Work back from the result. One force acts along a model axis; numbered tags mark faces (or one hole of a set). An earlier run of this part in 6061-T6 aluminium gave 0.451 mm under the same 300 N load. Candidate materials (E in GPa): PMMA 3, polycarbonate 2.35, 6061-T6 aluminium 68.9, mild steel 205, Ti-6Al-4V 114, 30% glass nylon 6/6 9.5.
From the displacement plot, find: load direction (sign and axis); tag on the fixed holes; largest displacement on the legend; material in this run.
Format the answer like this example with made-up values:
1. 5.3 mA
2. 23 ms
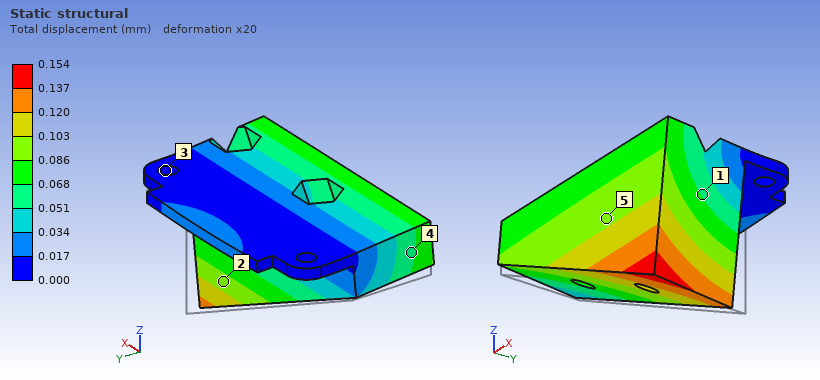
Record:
1. -Y
2. 3
3. 0.154 mm
4. mild steel
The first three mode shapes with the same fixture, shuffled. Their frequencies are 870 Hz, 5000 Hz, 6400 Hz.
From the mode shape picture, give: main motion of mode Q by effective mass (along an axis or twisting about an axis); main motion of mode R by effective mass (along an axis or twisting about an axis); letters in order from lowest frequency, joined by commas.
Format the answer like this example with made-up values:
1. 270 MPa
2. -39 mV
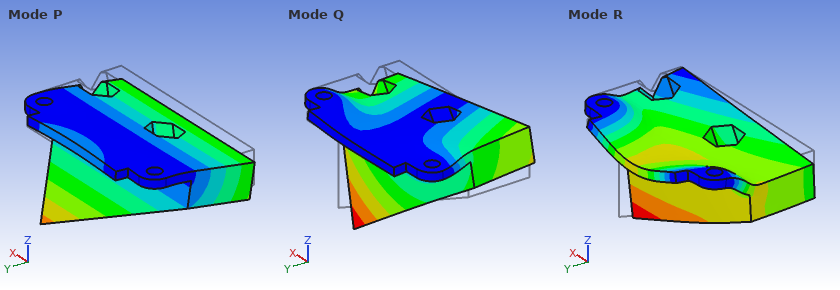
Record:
1. along X
2. along Z
3. P, Q, R
